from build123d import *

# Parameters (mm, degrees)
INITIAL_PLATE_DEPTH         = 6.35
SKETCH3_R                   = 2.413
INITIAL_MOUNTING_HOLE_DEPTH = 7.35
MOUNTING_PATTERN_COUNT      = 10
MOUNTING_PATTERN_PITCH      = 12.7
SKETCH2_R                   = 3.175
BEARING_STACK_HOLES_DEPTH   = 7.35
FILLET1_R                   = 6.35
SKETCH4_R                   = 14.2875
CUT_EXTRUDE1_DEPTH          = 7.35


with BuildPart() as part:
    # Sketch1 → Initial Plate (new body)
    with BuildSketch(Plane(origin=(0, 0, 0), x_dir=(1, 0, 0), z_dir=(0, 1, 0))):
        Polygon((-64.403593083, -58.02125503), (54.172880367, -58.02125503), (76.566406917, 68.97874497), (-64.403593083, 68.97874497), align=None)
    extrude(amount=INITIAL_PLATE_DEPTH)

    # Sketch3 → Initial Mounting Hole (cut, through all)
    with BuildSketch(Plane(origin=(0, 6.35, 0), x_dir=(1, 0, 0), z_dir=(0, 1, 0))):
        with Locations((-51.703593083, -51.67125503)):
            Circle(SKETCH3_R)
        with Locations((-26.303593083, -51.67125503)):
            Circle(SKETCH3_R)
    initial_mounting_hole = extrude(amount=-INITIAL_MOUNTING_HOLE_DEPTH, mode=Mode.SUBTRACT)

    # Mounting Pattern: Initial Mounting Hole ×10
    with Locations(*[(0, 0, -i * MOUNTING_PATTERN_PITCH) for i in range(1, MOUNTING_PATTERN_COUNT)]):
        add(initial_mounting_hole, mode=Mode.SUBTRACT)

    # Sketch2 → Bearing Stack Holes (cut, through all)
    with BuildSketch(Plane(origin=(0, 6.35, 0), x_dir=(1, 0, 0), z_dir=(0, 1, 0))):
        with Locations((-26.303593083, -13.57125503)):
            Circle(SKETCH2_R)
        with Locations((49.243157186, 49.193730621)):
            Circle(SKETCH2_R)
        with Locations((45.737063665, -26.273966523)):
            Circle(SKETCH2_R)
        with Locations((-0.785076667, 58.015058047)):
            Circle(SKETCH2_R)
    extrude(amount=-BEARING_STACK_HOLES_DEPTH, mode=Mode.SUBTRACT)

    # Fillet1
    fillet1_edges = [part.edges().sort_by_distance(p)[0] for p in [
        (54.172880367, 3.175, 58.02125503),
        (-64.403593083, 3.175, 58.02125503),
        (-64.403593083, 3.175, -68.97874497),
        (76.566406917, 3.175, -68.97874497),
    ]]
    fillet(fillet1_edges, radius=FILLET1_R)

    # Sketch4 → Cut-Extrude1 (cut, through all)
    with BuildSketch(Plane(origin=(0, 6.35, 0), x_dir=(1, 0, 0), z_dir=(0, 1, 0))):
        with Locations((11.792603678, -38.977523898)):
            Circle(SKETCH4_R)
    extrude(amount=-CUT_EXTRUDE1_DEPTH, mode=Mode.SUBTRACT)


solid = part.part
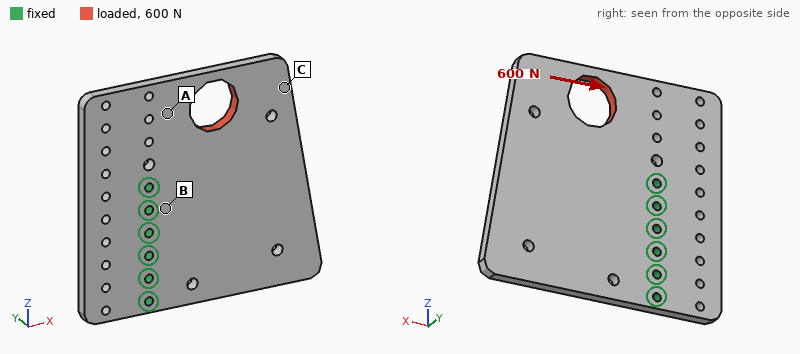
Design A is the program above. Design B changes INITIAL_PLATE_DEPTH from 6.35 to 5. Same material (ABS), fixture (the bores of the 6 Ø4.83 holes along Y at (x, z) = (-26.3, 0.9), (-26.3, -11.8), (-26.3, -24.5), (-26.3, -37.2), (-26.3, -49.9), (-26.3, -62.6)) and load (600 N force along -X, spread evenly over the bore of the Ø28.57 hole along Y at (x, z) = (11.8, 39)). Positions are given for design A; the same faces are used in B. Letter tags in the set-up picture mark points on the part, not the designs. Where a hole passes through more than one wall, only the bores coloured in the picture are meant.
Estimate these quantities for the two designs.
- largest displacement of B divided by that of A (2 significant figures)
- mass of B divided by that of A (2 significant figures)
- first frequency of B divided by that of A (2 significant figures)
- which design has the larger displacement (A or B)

1.3
0.79
0.79
B
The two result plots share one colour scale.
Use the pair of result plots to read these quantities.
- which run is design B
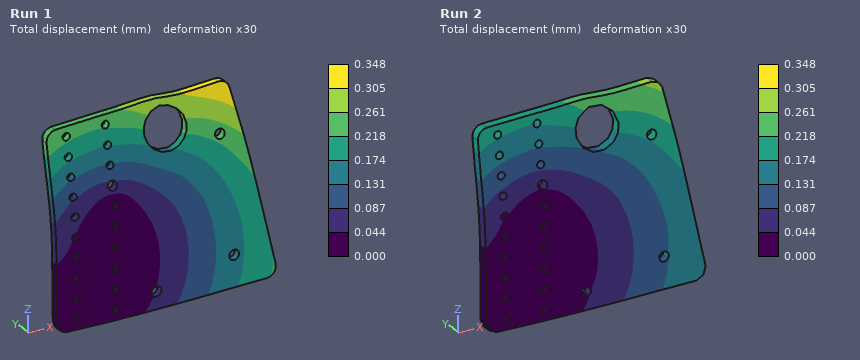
Run 1
